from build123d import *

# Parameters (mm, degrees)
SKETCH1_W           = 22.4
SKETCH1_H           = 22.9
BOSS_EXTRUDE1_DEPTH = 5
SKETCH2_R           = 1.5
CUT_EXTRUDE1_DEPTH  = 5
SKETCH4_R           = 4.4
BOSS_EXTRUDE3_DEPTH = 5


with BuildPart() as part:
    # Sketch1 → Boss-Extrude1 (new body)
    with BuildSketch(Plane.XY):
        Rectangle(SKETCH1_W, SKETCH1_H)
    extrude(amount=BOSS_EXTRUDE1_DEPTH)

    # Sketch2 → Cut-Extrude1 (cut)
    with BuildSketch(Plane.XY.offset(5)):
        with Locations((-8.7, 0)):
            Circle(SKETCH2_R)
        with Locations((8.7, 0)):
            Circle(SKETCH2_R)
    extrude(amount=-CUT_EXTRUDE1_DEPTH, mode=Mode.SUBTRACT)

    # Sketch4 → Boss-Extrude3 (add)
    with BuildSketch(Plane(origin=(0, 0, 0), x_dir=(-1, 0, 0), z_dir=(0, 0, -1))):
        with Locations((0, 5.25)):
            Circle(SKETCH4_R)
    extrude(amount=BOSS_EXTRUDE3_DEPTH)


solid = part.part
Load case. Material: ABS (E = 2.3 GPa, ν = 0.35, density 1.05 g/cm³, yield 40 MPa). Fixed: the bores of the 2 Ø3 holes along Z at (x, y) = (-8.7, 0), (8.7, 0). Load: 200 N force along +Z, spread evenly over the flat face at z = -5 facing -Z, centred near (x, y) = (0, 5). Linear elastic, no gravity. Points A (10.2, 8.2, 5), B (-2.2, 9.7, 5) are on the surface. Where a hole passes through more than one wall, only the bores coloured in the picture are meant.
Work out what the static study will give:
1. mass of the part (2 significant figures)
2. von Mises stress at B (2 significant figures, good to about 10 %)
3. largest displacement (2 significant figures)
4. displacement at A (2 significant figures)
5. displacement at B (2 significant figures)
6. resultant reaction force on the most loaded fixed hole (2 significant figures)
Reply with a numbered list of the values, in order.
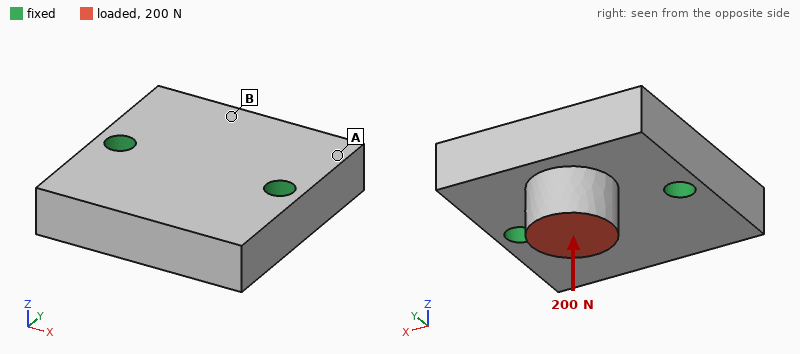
1. 2.9 g
2. 4.8 MPa
3. 0.12 mm
4. 0.052 mm
5. 0.094 mm
6. 100 N
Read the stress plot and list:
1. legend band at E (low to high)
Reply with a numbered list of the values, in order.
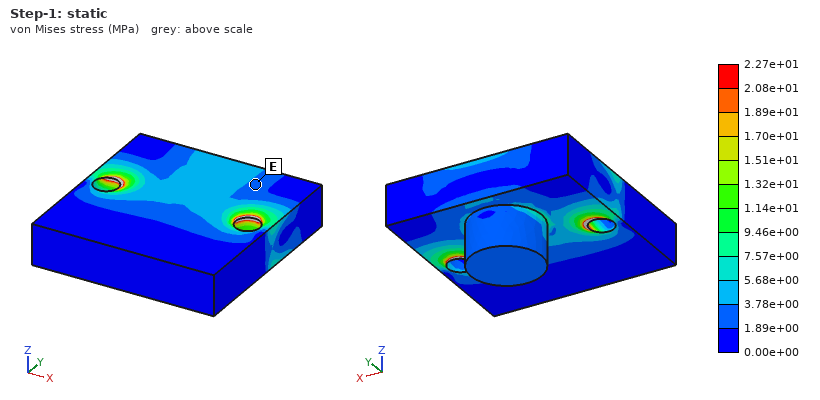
1. 1.89e+00 to 3.78e+00 MPa
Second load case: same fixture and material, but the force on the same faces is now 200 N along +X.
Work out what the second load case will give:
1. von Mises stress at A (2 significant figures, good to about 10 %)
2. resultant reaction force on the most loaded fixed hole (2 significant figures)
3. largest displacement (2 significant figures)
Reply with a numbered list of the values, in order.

1. 1.6 MPa
2. 150 N
3. 0.10 mm
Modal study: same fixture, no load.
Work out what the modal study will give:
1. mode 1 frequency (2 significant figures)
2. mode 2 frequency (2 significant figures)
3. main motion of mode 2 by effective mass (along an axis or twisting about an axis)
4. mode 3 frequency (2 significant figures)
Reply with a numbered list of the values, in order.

1. 6100 Hz
2. 8100 Hz
3. along Z
4. 12 kHz
